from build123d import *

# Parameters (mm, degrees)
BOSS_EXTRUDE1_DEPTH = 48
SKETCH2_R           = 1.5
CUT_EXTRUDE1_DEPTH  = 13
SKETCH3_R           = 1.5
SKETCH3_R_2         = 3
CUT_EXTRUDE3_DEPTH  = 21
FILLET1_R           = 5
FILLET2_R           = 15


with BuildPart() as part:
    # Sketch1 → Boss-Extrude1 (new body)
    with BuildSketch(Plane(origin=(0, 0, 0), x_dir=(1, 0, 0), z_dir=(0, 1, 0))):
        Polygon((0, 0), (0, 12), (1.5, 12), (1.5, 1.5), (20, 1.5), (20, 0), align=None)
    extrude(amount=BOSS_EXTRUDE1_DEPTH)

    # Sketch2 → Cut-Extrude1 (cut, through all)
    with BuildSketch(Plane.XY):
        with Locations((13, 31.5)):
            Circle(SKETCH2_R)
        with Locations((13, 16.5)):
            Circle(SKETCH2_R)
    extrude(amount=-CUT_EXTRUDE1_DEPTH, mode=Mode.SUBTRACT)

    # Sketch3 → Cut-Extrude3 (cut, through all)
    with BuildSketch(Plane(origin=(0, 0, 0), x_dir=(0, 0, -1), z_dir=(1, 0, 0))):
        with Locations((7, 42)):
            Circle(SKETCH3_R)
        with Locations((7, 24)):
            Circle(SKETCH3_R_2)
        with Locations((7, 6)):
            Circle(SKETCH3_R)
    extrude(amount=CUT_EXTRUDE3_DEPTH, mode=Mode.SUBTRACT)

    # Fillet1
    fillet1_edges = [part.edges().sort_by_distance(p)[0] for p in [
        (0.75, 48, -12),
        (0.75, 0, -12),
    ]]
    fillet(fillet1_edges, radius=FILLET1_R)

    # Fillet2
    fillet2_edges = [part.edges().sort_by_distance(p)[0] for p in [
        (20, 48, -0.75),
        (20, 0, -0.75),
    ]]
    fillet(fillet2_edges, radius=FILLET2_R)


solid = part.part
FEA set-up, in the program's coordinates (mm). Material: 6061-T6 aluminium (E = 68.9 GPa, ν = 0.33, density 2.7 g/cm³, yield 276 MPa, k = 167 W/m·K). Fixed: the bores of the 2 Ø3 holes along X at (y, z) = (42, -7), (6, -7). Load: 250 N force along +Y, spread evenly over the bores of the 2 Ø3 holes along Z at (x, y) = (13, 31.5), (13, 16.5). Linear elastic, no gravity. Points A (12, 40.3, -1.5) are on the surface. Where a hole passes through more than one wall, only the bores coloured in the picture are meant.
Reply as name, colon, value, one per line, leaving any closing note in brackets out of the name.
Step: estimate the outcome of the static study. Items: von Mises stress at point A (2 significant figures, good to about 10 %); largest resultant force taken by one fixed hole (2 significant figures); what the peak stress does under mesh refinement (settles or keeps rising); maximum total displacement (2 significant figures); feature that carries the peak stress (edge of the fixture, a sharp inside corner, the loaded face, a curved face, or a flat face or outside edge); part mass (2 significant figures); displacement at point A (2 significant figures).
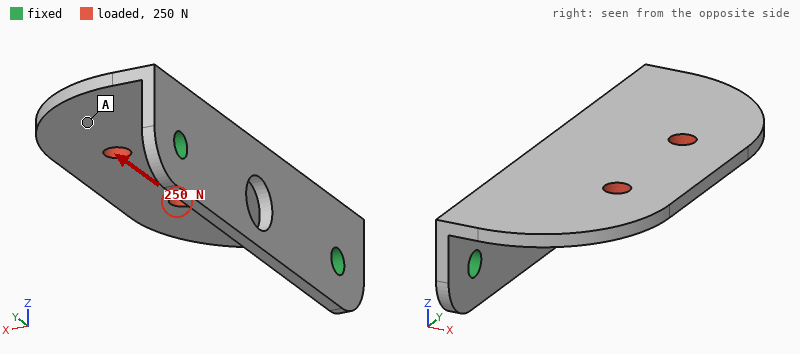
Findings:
von Mises stress at point A: 10 MPa
largest resultant force taken by one fixed hole: 150 N
what the peak stress does under mesh refinement: keeps rising
maximum total displacement: 43 µm
feature that carries the peak stress: edge of the fixture
part mass: 5.3 g
displacement at point A: 31 µm
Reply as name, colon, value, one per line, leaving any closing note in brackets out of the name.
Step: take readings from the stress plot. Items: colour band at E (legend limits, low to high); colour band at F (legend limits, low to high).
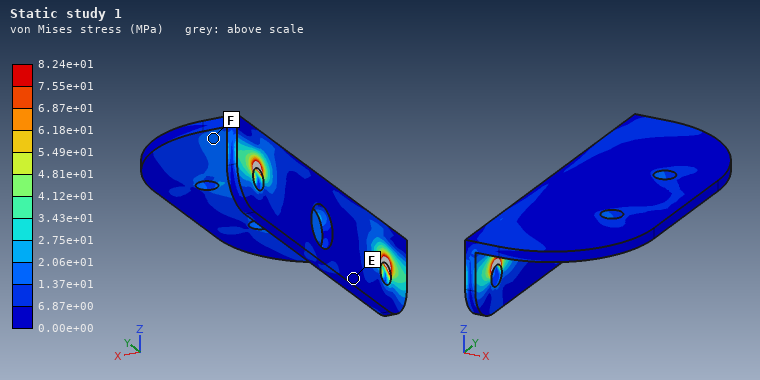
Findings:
colour band at E: 0.00e+00 to 6.87e+00 MPa
colour band at F: 1.37e+01 to 2.06e+01 MPa
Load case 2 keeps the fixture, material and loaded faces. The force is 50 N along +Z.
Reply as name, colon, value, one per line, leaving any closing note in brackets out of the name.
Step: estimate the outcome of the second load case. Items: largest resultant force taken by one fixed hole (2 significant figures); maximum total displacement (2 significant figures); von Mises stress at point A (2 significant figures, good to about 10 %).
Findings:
largest resultant force taken by one fixed hole: 28 N
maximum total displacement: 0.18 mm
von Mises stress at point A: 10 MPa
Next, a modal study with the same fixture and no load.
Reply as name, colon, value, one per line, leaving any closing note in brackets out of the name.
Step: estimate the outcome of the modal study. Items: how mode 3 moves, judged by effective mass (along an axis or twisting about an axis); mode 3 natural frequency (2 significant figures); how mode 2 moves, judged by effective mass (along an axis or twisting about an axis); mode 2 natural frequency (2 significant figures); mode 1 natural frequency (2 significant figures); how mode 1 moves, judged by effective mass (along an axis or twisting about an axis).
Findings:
how mode 3 moves, judged by effective mass: along X
mode 3 natural frequency: 7900 Hz
how mode 2 moves, judged by effective mass: twisting about X
mode 2 natural frequency: 4600 Hz
mode 1 natural frequency: 2300 Hz
how mode 1 moves, judged by effective mass: along Z
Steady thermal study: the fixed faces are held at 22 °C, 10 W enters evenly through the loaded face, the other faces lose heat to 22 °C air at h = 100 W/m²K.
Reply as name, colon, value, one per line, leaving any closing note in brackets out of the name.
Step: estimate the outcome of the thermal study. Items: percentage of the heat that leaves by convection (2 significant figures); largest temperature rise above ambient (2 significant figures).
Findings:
percentage of the heat that leaves by convection: 28 %
largest temperature rise above ambient: 21 K
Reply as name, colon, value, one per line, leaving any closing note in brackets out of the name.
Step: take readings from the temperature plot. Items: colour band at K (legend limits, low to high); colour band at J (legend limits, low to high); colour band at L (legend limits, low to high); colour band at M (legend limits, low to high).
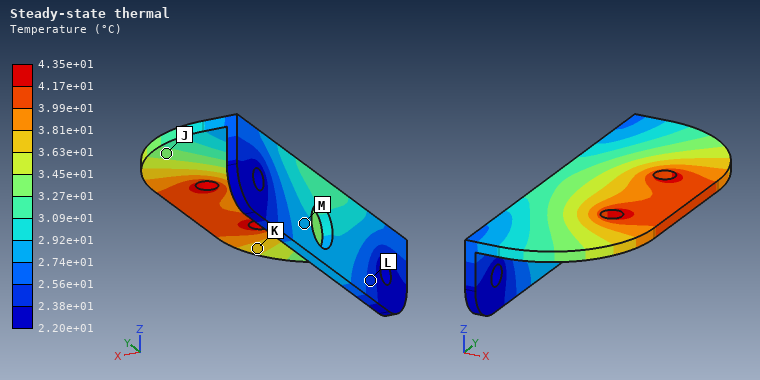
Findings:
colour band at K: 3.63e+01 to 3.81e+01 °C
colour band at J: 3.27e+01 to 3.45e+01 °C
colour band at L: 2.38e+01 to 2.56e+01 °C
colour band at M: 2.74e+01 to 2.92e+01 °C
